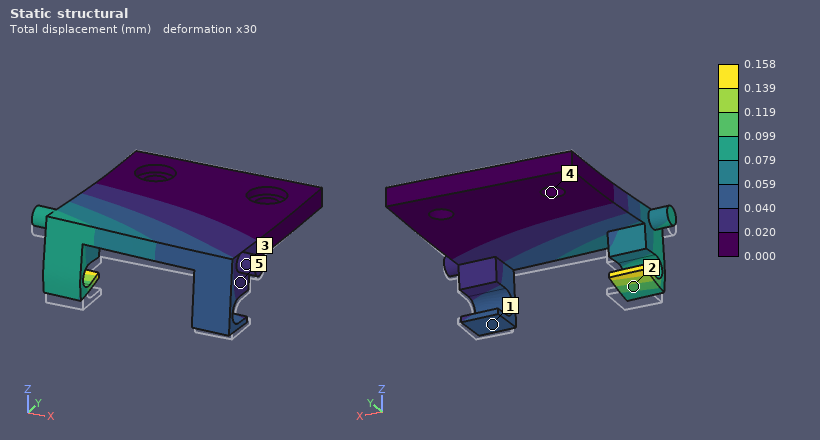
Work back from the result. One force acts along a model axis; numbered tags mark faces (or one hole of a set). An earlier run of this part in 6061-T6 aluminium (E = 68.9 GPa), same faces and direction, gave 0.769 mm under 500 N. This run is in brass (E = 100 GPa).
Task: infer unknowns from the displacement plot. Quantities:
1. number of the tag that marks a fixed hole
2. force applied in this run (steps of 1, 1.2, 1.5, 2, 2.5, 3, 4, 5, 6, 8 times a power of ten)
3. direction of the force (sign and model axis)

4
150 N
+Z
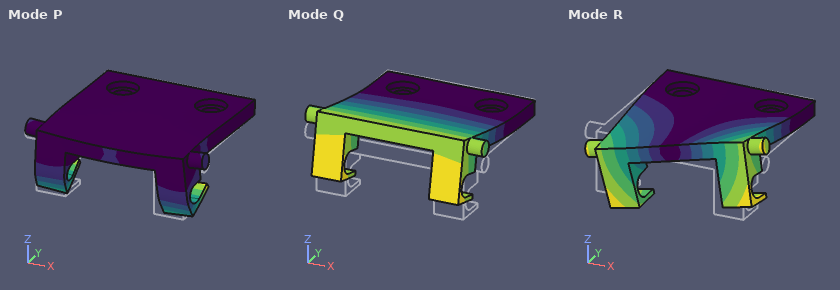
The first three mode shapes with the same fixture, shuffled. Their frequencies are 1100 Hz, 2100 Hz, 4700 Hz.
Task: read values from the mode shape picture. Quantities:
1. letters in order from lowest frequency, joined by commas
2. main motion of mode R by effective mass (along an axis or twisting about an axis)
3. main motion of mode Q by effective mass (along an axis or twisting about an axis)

Q, R, P
twisting about Y
along Z
